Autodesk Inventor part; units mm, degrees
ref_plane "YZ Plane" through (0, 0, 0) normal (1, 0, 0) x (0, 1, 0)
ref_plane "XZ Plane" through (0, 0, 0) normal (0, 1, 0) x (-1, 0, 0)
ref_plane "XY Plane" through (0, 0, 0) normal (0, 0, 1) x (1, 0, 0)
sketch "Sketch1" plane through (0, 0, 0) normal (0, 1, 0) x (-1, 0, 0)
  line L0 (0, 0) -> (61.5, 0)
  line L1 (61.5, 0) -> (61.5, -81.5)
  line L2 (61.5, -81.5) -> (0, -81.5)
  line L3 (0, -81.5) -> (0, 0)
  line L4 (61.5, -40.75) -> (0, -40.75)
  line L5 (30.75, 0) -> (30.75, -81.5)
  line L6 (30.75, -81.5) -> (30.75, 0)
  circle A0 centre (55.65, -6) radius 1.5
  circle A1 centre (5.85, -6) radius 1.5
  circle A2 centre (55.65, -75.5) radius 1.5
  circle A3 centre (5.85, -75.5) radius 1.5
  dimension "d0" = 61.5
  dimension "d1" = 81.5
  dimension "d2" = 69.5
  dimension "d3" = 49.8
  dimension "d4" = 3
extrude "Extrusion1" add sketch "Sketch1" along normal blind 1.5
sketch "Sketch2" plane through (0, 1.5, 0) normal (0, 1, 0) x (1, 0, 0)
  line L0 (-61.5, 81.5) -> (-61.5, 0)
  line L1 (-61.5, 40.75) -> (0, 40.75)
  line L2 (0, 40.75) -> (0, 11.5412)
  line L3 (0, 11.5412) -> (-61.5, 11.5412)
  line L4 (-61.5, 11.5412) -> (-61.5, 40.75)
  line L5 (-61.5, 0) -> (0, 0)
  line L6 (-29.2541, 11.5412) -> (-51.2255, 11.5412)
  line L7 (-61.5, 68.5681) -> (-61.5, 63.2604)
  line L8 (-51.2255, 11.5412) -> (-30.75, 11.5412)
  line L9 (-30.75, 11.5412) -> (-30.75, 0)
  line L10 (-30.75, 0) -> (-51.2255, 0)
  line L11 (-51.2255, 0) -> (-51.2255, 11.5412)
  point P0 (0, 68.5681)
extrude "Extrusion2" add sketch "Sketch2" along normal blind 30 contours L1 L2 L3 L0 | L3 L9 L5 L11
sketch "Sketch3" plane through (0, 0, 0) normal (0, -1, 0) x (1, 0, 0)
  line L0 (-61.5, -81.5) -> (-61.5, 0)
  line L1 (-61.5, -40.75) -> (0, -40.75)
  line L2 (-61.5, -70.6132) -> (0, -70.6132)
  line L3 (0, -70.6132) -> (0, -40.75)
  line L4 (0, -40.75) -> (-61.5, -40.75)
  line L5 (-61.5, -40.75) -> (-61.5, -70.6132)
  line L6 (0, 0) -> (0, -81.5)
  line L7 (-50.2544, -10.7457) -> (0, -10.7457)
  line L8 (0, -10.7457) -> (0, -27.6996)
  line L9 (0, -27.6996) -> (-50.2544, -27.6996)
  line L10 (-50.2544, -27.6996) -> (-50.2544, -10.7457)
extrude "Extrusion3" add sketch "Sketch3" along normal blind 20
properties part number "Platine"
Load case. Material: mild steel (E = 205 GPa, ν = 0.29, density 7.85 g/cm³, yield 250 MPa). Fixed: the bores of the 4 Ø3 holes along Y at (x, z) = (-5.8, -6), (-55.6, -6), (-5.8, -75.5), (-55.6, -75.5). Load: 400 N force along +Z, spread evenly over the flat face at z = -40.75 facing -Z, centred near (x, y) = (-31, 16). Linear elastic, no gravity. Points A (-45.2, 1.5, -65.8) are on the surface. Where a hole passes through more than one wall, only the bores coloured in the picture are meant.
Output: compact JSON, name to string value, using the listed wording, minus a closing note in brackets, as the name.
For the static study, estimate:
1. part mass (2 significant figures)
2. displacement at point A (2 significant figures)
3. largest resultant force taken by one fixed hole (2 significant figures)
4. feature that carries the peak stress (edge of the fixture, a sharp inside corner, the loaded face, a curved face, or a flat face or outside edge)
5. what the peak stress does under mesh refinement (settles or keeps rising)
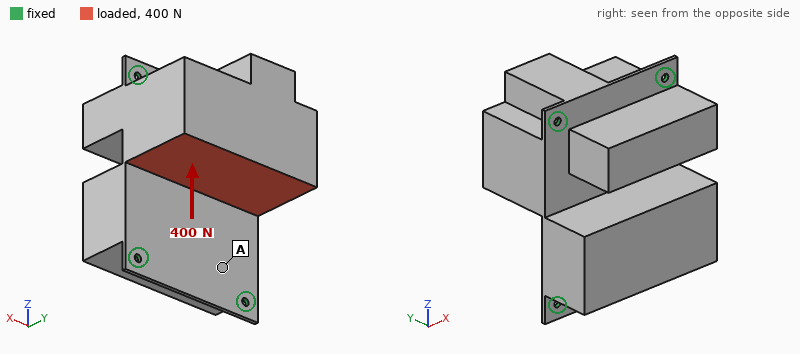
{"part mass": "960 g", "displacement at point A": "3.5 µm", "largest resultant force taken by one fixed hole": "150 N", "feature that carries the peak stress": "edge of the fixture", "what the peak stress does under mesh refinement": "keeps rising"}
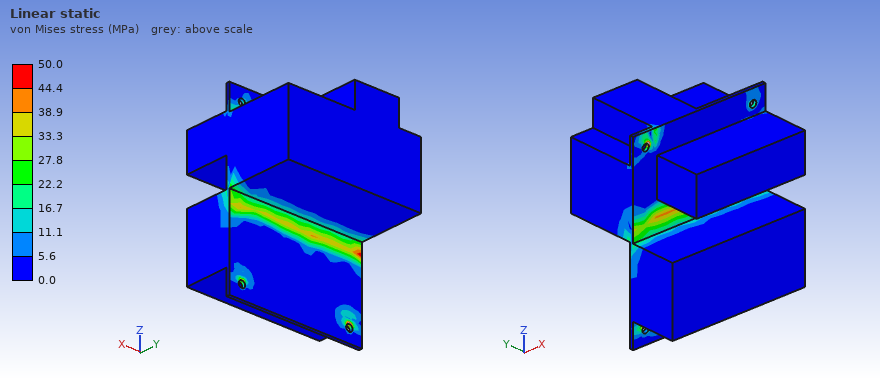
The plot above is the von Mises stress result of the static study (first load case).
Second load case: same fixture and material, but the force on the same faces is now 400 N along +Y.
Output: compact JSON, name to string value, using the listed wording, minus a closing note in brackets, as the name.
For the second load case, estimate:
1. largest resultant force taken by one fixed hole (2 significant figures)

{"largest resultant force taken by one fixed hole": "110 N"}
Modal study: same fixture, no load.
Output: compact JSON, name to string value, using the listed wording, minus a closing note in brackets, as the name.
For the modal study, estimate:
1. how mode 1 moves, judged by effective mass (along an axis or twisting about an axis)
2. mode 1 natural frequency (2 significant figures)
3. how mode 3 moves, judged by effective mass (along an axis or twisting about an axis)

{"how mode 1 moves, judged by effective mass": "along Y", "mode 1 natural frequency": "890 Hz", "how mode 3 moves, judged by effective mass": "along Y"}
